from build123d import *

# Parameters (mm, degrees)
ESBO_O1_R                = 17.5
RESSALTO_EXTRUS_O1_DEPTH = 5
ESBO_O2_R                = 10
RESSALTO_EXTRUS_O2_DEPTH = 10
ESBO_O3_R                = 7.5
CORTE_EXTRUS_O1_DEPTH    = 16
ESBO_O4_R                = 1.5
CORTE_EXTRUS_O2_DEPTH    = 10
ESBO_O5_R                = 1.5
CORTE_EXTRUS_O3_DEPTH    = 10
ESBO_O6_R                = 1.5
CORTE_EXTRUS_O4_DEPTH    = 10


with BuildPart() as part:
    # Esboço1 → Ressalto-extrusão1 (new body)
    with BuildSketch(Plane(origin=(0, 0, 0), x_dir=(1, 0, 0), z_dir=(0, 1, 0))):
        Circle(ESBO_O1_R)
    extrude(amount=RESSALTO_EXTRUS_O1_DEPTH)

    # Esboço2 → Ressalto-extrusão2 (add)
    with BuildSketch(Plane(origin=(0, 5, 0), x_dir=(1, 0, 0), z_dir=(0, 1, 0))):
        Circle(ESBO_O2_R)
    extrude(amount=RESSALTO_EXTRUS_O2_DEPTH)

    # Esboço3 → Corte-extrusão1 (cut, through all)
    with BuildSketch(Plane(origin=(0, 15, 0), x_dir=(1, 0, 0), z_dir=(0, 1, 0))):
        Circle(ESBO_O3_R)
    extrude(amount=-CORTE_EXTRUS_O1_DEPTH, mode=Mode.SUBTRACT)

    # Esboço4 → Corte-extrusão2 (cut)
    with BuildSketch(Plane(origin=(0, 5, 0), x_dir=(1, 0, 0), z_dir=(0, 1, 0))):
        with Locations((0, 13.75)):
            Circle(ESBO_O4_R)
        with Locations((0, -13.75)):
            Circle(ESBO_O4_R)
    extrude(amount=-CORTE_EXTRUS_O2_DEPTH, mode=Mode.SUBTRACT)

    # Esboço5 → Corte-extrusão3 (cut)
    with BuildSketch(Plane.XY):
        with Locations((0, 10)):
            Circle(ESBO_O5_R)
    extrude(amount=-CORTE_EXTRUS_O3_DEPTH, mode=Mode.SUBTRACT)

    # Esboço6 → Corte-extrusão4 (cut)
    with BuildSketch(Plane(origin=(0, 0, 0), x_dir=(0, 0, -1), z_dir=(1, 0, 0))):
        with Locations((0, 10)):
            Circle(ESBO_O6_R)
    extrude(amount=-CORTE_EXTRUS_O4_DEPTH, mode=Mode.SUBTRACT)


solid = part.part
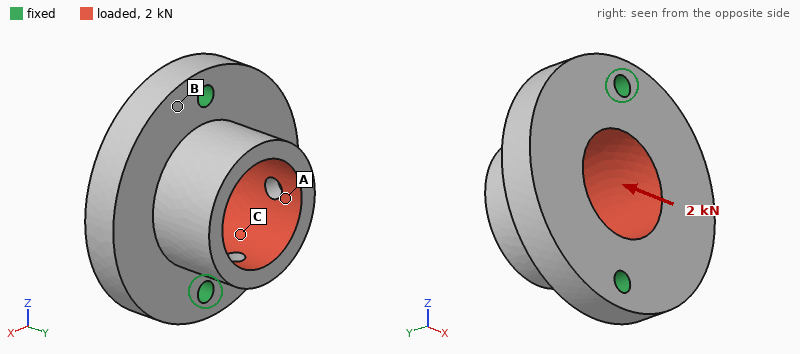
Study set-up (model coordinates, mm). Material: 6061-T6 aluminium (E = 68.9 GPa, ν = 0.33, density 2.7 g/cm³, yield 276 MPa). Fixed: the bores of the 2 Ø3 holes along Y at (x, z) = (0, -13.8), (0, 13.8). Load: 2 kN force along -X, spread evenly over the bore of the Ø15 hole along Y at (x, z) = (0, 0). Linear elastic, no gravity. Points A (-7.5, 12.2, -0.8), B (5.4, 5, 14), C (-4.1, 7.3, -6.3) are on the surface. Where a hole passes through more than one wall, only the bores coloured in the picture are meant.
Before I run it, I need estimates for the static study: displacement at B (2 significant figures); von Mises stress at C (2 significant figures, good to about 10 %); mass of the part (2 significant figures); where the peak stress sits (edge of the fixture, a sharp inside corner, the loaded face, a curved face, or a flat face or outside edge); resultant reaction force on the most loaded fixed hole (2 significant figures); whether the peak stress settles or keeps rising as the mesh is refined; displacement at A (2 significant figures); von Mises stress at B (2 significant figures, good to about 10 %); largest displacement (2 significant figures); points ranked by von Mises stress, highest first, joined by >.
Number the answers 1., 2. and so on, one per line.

1. 7.1 µm
2. 24 MPa
3. 14 g
4. edge of the fixture
5. 1.0 kN
6. keeps rising
7. 32 µm
8. 43 MPa
9. 41 µm
10. B > C > A
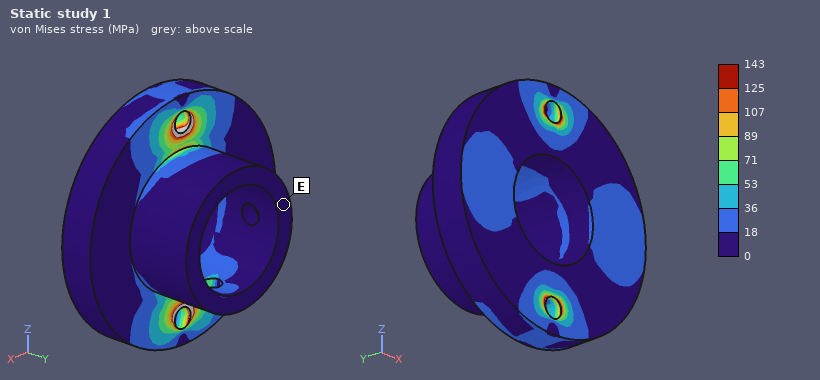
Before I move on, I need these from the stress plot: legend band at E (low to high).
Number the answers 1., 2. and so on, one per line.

1. 0 to 18 MPa
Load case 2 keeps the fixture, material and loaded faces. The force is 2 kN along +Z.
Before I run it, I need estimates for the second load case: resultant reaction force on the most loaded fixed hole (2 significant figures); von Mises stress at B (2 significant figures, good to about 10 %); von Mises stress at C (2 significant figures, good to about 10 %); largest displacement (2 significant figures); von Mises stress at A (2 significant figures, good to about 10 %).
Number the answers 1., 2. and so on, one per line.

1. 1.1 kN
2. 9.8 MPa
3. 20 MPa
4. 11 µm
5. 21 MPa
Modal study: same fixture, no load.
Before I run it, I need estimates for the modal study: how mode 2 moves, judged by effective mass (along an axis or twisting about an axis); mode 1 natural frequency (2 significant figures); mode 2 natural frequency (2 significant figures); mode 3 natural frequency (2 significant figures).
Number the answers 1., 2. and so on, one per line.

1. along Y
2. 9700 Hz
3. 15 kHz
4. 27 kHz
